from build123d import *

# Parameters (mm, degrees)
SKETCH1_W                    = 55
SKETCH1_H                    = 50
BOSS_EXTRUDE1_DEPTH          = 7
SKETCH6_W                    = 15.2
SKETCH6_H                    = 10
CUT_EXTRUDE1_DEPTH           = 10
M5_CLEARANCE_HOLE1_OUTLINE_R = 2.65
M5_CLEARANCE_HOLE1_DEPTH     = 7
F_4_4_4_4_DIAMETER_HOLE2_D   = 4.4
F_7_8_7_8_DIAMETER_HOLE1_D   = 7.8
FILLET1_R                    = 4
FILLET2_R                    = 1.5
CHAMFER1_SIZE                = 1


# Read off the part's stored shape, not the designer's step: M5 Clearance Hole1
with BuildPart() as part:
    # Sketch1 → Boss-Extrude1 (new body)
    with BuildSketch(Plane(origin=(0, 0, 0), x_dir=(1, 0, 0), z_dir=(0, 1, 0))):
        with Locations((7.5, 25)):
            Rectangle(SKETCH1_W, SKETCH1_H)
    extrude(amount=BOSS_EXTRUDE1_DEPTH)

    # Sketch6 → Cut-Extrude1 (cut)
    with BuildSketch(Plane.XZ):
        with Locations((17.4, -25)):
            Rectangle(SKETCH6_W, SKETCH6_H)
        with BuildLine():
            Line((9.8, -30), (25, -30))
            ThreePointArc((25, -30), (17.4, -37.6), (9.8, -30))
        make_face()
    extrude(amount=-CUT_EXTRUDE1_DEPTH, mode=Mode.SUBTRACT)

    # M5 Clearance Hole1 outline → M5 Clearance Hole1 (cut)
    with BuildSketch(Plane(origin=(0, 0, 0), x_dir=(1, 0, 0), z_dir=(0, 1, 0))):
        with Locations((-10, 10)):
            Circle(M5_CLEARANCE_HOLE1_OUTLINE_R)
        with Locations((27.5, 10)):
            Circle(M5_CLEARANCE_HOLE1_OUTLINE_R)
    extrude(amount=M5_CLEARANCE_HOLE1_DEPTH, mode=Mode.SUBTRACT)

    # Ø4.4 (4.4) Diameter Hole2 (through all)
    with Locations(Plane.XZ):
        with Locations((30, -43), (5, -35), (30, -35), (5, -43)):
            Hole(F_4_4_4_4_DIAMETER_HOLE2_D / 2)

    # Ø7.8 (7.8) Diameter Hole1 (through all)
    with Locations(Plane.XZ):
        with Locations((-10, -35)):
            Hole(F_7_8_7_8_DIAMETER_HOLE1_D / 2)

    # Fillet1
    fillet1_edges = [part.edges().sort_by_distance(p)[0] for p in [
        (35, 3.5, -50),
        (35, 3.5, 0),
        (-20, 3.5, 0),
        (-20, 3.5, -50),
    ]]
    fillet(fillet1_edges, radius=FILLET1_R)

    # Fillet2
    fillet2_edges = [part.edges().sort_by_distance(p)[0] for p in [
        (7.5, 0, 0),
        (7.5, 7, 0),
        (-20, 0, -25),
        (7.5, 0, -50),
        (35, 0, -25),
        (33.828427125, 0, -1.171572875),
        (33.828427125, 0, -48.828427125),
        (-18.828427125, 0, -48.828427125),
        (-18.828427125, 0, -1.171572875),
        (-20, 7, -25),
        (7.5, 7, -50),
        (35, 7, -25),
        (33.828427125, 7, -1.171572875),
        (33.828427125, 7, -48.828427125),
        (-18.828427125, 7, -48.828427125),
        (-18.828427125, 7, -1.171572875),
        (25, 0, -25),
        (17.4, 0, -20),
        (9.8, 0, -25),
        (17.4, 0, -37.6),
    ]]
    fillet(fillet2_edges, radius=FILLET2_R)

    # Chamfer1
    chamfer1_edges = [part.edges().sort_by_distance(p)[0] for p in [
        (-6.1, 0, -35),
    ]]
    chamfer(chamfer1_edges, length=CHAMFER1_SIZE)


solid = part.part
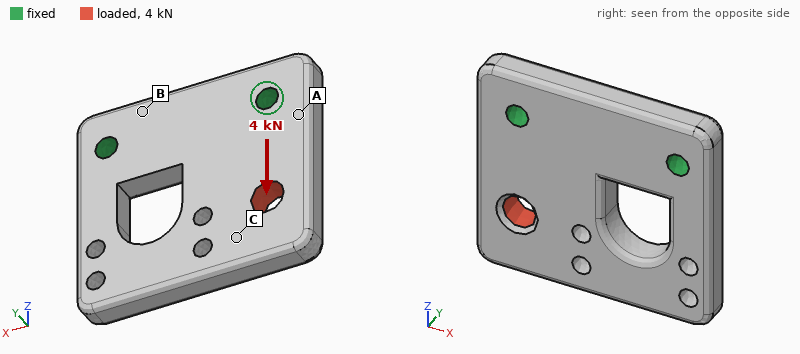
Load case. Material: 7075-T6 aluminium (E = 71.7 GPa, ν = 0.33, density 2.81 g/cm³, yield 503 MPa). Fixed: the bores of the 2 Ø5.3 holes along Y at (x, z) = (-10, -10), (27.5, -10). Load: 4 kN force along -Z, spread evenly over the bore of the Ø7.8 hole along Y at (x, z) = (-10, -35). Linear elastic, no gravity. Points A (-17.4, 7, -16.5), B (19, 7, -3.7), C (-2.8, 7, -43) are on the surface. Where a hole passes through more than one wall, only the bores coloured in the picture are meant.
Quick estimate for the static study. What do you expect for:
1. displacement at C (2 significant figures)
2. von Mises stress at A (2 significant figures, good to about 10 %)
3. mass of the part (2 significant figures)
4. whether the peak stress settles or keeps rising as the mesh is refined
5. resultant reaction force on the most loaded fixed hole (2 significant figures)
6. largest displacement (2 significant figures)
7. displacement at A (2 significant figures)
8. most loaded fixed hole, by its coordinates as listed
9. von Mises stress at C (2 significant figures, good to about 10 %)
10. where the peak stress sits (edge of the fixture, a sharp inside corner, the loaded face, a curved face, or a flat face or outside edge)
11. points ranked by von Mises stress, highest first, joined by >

19 µm
30 MPa
45 g
keeps rising
3.9 kN
27 µm
6.1 µm
(-10, -10)
17 MPa
edge of the fixture
A > C > B
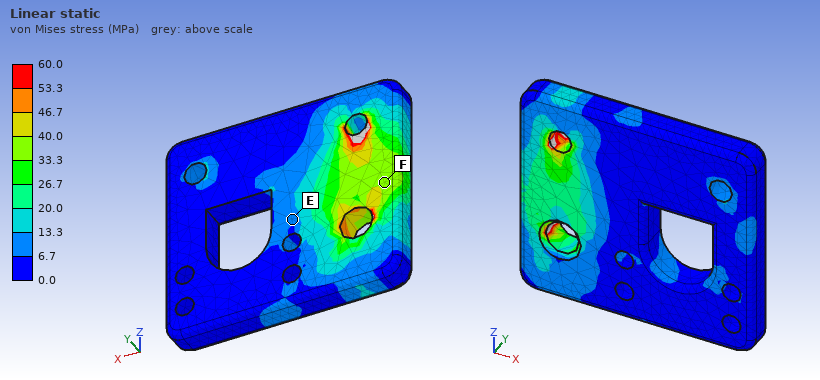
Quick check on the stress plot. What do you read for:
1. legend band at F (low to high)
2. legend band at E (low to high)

33.3 to 40.0 MPa
6.7 to 13.3 MPa
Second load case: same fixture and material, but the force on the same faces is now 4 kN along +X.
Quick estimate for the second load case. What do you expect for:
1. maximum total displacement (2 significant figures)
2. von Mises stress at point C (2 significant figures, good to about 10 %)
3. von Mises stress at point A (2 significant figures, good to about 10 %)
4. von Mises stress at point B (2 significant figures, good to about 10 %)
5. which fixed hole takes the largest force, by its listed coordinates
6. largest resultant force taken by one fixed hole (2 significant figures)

42 µm
20 MPa
22 MPa
11 MPa
(-10, -10)
3.4 kN
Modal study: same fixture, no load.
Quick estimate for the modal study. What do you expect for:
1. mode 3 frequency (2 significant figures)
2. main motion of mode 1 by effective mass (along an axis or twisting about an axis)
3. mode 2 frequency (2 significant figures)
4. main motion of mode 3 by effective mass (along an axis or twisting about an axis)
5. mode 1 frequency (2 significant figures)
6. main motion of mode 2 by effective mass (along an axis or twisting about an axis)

11 kHz
along Y
6100 Hz
along X
3200 Hz
twisting about Z
